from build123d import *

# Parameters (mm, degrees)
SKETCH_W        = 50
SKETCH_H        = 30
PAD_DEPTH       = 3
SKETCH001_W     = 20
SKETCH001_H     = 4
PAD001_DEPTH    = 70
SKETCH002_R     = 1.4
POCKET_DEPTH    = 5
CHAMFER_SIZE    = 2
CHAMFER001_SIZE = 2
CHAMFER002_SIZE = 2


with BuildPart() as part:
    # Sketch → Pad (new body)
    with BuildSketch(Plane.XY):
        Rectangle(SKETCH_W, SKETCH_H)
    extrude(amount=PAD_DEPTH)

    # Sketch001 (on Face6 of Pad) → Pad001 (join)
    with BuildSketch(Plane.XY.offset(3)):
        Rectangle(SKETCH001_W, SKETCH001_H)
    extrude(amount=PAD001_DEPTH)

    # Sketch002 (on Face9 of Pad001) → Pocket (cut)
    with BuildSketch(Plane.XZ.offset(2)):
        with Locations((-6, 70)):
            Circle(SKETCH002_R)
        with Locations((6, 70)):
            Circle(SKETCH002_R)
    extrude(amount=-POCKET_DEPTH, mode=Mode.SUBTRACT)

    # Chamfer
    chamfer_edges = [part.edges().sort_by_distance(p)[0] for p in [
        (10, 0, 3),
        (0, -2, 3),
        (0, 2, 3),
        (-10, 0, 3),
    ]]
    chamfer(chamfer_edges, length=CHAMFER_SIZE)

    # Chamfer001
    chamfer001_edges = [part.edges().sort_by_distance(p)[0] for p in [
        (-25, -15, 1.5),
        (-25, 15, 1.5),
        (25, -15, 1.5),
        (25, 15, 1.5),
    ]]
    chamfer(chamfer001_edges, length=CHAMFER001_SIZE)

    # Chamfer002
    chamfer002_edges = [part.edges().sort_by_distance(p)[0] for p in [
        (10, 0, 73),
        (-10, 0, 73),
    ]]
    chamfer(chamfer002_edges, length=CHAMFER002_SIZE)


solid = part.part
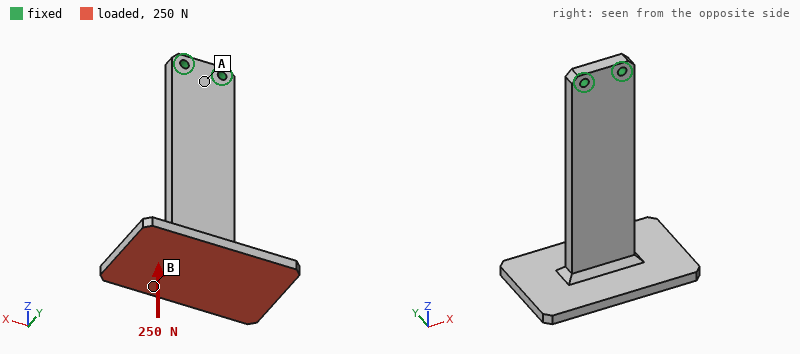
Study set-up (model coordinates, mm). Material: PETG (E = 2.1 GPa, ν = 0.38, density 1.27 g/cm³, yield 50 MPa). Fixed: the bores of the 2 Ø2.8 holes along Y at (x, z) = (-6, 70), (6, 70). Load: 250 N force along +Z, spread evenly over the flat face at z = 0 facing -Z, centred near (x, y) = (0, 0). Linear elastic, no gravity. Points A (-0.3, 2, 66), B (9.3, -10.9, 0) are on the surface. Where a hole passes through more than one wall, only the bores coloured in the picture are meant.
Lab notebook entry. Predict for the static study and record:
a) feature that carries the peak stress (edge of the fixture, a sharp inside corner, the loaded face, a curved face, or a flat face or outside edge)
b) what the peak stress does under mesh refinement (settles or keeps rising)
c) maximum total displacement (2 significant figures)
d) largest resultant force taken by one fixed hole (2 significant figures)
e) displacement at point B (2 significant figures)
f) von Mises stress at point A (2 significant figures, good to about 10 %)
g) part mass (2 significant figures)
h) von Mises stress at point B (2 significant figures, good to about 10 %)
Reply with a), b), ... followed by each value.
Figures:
a) a sharp inside corner
b) keeps rising
c) 0.54 mm
d) 130 N
e) 0.19 mm
f) 1.8 MPa
g) 13 g
h) 5.8 MPa
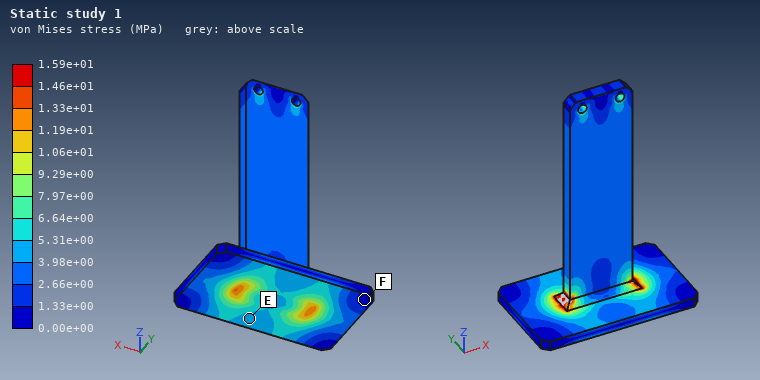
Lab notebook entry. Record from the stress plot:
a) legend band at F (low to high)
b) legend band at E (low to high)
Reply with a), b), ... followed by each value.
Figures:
a) 0.00e+00 to 1.33e+00 MPa
b) 3.98e+00 to 5.31e+00 MPa
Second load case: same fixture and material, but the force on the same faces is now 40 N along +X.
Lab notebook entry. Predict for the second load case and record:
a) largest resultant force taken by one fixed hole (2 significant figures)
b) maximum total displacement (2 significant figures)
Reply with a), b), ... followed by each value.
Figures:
a) 210 N
b) 1.0 mm
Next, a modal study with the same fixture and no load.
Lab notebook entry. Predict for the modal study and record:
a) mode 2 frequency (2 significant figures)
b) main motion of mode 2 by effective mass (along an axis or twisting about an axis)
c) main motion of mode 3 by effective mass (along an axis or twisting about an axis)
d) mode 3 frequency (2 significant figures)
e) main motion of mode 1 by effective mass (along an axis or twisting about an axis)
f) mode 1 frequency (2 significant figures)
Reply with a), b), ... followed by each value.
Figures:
a) 270 Hz
b) twisting about Z
c) along X
d) 390 Hz
e) along Y
f) 85 Hz
